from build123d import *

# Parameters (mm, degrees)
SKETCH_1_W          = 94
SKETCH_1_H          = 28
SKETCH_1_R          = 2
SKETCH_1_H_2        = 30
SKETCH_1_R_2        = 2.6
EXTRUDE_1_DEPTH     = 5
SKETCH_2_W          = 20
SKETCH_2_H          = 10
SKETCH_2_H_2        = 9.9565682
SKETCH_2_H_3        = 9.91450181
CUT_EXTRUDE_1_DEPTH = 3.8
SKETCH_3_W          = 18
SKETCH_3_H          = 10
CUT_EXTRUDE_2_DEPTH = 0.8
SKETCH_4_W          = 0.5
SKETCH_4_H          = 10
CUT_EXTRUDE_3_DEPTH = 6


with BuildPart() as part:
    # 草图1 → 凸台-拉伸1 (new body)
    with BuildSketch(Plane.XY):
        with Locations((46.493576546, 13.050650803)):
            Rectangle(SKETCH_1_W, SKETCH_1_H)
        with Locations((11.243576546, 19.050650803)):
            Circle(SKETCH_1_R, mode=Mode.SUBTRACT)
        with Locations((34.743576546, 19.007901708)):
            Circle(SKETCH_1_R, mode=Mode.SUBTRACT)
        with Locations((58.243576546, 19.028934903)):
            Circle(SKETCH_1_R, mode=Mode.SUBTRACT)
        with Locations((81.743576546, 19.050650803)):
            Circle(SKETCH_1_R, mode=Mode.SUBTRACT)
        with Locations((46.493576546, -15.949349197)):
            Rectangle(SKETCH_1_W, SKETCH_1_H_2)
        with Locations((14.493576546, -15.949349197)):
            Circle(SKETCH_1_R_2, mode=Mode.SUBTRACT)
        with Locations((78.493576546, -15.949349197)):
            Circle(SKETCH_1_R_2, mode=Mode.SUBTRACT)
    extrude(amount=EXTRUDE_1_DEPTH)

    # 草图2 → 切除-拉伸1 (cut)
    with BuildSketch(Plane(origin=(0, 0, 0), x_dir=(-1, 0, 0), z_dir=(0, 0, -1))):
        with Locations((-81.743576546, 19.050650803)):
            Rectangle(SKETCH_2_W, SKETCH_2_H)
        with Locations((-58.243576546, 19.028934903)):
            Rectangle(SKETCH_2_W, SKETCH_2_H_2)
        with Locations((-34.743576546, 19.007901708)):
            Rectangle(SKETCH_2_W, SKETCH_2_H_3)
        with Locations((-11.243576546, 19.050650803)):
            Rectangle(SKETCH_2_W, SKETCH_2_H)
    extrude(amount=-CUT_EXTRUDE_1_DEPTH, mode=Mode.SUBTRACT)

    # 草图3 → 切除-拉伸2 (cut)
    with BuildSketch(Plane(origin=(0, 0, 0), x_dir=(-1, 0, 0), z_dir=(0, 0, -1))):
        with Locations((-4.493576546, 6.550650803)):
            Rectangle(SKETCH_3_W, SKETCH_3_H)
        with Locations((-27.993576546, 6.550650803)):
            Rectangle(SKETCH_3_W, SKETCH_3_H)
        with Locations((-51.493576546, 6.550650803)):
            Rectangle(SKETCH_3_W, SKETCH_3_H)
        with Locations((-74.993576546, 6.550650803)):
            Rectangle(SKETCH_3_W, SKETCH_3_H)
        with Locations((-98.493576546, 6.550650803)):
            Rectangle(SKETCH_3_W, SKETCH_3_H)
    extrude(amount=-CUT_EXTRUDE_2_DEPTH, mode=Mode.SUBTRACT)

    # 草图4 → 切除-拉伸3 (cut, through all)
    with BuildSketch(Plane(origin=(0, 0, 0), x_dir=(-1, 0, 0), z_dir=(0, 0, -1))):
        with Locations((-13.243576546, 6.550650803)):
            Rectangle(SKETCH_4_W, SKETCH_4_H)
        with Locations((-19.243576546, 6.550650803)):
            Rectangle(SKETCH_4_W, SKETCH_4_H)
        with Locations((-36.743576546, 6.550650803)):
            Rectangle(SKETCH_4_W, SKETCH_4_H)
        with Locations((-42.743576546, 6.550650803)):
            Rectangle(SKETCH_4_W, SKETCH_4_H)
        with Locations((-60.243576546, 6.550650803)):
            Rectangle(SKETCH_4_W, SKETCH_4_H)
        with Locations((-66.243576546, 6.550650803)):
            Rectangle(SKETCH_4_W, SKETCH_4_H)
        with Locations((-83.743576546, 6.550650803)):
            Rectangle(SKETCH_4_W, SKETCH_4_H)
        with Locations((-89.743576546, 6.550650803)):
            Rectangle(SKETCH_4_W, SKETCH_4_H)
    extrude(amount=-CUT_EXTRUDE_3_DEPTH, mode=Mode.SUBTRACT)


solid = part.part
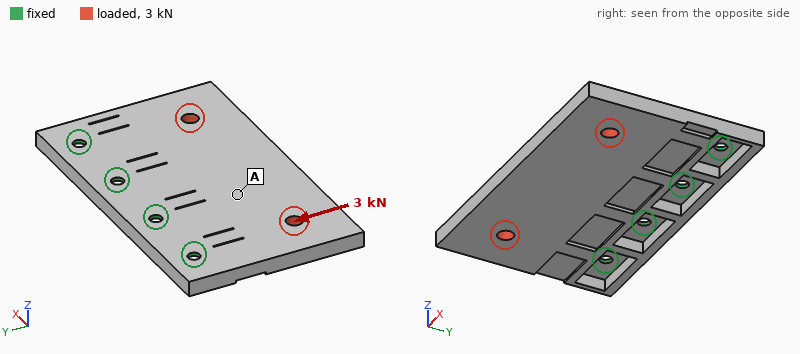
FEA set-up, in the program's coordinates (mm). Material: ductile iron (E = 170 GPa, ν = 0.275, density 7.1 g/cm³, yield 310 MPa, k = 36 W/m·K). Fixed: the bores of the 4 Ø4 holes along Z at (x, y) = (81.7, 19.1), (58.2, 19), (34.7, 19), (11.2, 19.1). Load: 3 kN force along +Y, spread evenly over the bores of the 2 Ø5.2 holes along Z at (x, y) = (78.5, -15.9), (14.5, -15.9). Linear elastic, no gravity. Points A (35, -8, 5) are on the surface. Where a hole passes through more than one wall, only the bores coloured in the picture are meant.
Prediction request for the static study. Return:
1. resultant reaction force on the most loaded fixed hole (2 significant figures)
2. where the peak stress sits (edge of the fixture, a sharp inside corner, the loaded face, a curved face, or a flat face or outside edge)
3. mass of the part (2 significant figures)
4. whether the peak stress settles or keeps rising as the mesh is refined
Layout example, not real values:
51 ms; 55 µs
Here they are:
820 N; edge of the fixture; 160 g; keeps rising
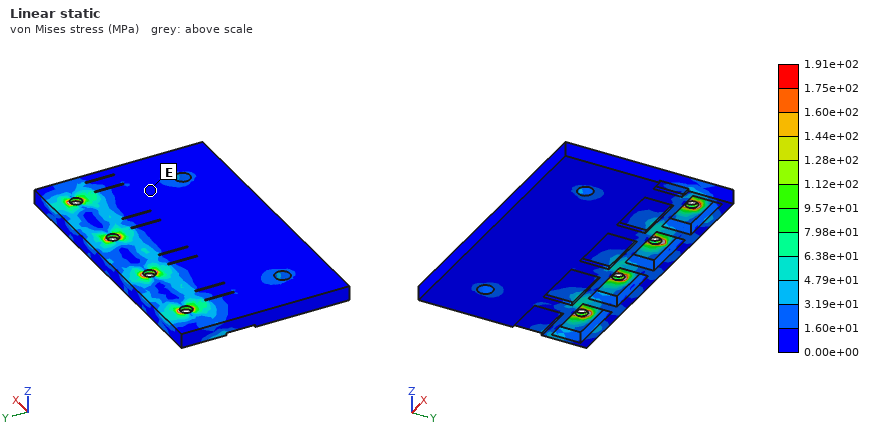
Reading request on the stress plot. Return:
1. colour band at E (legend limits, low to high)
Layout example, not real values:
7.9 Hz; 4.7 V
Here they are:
0.00e+00 to 1.60e+01 MPa
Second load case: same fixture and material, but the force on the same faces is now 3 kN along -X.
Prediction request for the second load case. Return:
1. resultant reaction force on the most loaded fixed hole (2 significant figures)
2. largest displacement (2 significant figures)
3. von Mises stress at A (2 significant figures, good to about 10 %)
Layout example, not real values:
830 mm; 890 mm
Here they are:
1.5 kN; 34 µm; 21 MPa
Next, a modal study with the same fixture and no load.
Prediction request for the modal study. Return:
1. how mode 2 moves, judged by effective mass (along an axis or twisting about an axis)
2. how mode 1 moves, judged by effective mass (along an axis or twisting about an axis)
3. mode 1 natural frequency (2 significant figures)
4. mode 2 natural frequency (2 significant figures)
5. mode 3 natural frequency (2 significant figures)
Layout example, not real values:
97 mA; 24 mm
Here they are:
twisting about Y; along Z; 530 Hz; 1500 Hz; 3800 Hz
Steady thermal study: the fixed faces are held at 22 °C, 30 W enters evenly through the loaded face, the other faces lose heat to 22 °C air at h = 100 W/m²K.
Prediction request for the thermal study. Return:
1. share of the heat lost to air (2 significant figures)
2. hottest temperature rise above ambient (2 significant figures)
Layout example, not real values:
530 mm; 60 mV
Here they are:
83 %; 52 K
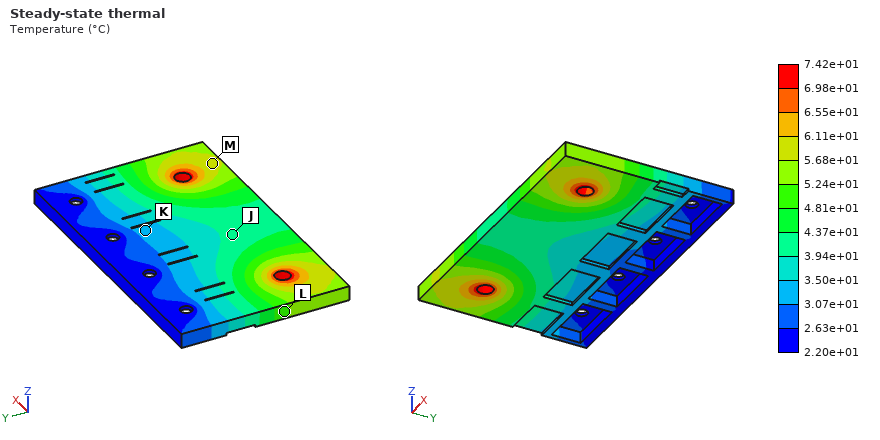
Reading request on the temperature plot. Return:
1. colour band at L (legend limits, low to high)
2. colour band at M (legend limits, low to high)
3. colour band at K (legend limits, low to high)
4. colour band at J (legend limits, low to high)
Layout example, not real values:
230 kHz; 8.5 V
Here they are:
4.81e+01 to 5.24e+01 °C; 5.68e+01 to 6.11e+01 °C; 3.07e+01 to 3.50e+01 °C; 3.94e+01 to 4.37e+01 °C
